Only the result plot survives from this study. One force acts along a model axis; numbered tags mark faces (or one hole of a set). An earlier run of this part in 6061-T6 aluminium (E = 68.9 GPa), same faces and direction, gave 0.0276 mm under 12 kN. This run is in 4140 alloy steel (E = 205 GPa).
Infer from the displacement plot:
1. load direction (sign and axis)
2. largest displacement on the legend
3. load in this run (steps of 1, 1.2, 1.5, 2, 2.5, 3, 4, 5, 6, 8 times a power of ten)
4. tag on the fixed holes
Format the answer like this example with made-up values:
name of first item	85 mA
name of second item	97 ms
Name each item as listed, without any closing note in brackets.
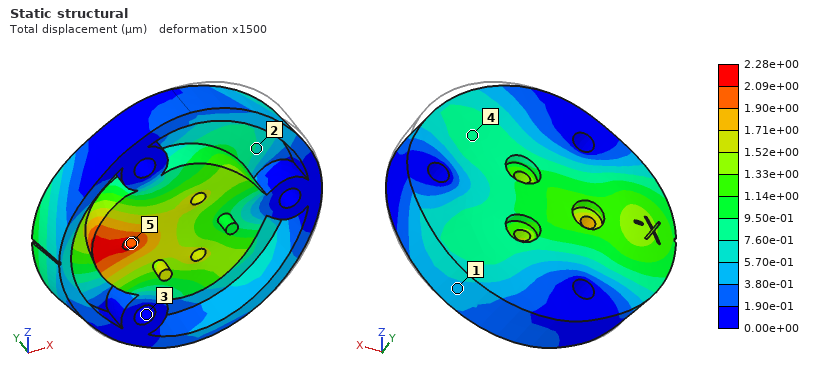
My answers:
load direction	-X
largest displacement on the legend	2.28e+00 µm
load in this run	3 kN
tag on the fixed holes	3
